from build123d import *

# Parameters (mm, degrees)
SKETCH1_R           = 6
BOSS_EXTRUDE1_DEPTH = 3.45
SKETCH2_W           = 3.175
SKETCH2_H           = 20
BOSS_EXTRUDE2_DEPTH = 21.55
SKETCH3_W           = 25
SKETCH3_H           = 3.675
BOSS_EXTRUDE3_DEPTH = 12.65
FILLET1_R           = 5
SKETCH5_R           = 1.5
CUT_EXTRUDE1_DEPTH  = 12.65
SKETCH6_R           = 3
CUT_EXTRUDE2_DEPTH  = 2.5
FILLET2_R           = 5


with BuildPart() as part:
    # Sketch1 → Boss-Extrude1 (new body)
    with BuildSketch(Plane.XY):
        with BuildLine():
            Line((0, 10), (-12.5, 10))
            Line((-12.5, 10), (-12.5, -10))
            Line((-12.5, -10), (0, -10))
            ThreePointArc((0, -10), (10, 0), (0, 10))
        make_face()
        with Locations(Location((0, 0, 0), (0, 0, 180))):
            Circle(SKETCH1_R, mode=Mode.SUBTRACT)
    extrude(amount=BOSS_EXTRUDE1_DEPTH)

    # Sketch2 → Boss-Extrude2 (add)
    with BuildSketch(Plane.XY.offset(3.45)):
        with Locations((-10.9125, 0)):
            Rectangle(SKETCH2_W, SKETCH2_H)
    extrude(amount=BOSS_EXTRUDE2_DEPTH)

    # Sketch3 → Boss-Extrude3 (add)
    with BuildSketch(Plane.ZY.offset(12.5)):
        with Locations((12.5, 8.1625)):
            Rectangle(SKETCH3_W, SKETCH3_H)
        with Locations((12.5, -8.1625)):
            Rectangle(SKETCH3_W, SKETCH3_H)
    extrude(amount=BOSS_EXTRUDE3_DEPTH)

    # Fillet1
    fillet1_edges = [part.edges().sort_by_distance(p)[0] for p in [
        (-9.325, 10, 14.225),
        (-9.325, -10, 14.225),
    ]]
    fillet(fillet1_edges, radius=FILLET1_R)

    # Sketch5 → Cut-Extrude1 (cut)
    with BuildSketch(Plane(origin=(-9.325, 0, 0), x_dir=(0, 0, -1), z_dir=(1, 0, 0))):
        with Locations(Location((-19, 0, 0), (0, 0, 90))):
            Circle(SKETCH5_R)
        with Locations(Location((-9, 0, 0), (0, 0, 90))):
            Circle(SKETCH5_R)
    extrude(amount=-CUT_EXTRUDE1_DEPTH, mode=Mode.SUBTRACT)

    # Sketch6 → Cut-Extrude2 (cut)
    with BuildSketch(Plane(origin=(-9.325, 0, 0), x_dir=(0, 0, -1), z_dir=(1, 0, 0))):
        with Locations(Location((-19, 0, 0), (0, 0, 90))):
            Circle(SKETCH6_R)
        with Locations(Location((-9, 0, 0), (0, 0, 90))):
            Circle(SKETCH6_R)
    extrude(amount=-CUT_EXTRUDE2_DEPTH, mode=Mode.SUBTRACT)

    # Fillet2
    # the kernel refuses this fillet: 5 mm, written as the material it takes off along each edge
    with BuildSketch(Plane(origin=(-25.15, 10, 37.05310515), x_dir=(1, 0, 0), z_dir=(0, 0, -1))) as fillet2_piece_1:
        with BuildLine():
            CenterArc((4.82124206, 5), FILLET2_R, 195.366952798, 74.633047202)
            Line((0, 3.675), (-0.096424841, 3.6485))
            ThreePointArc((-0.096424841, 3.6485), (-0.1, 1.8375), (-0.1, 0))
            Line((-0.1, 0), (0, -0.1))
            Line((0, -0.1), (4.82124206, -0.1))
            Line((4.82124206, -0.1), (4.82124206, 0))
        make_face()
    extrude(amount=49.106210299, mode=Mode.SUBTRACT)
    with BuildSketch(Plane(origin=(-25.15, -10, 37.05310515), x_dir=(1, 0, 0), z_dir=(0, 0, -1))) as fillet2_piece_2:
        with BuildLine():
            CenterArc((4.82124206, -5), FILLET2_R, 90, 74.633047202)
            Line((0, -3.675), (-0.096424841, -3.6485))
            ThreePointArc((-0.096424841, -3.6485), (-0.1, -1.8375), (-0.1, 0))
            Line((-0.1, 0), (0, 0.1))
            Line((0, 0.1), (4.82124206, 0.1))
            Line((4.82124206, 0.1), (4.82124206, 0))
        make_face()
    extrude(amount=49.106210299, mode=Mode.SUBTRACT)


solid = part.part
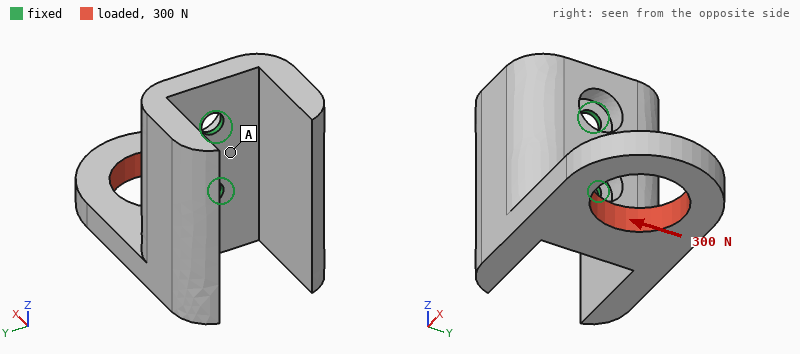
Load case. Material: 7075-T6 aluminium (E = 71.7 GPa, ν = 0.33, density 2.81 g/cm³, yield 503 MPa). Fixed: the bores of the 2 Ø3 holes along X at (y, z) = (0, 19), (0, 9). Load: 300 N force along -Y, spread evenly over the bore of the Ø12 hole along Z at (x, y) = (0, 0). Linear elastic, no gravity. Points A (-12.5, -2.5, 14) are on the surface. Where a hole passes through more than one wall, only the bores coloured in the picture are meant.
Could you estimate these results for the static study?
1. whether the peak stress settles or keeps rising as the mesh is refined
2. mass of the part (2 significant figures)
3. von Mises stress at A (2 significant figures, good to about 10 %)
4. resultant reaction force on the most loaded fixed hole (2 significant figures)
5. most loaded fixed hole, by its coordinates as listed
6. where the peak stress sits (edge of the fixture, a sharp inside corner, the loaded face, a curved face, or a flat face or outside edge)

keeps rising
12 g
81 MPa
440 N
(0, 9)
edge of the fixture
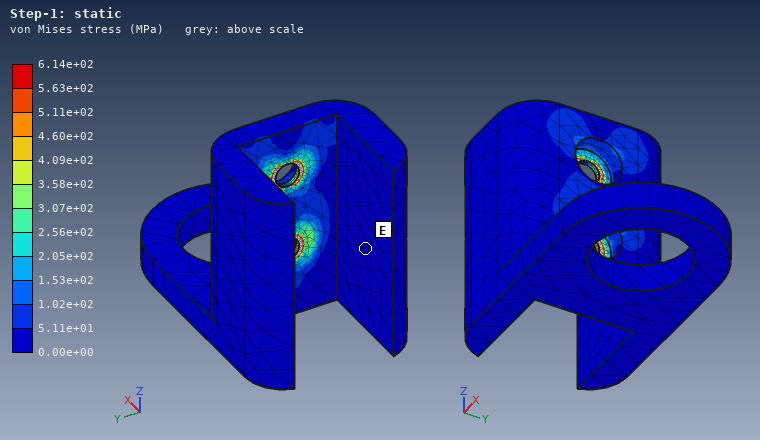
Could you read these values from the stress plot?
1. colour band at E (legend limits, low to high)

0.00e+00 to 5.11e+01 MPa
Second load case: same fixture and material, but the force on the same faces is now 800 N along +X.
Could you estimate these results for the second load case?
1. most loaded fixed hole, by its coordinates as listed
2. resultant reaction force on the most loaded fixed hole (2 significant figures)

(0, 9)
1.3 kN
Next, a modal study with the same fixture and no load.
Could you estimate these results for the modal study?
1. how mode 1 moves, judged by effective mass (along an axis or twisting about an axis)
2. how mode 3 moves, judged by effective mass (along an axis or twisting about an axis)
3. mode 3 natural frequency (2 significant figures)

twisting about Z
along Y
7000 Hz
